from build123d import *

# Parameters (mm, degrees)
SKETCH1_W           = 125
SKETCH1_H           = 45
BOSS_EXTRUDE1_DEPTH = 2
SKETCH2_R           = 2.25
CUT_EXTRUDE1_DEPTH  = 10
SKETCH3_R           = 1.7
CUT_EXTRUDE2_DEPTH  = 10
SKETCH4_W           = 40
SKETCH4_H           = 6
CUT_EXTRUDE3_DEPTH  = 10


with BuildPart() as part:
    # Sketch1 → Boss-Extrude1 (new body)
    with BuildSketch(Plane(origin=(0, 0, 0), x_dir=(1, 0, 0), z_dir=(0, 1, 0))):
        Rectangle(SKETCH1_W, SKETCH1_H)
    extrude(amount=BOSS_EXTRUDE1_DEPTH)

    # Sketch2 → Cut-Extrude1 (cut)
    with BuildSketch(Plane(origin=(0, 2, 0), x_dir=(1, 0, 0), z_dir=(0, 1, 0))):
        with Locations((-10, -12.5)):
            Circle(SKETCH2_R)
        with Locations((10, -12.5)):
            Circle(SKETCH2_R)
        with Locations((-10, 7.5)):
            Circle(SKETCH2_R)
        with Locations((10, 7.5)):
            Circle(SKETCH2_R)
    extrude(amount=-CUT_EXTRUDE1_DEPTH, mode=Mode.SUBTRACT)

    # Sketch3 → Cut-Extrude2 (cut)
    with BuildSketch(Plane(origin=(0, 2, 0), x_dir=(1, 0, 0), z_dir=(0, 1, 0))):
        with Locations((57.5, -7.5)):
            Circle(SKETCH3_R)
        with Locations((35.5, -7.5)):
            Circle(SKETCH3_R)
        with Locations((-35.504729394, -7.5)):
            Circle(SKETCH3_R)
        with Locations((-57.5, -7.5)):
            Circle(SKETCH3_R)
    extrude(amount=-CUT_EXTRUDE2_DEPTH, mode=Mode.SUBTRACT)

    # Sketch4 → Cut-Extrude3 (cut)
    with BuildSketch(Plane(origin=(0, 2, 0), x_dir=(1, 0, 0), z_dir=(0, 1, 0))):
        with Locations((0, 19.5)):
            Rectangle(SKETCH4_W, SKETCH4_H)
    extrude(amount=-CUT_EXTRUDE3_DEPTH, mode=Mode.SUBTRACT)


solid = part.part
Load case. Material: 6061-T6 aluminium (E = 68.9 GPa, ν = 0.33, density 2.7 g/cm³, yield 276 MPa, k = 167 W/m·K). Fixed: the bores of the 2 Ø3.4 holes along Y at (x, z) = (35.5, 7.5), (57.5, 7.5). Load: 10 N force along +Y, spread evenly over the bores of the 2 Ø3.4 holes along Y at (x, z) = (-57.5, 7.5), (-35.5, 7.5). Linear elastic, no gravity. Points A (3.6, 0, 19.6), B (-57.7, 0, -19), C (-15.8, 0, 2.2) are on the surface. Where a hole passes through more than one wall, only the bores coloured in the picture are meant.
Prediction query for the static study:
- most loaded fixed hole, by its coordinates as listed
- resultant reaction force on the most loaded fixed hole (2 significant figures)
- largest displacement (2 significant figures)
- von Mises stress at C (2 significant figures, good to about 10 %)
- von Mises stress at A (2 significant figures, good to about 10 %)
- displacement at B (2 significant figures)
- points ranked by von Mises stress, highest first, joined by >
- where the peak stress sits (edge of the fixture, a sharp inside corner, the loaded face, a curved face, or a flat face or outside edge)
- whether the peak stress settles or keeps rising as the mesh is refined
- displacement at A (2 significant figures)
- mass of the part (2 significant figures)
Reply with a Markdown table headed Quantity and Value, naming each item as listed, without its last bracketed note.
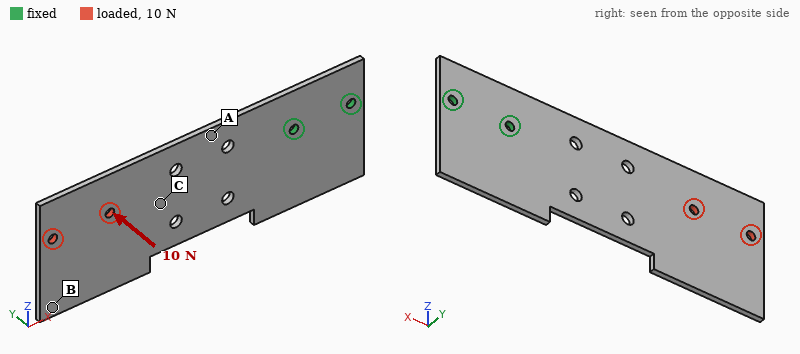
| Quantity | Value |
|---|---|
| most loaded fixed hole, by its coordinates as listed | (35.5, 7.5) |
| resultant reaction force on the most loaded fixed hole | 26 N |
| largest displacement | 1.4 mm |
| von Mises stress at C | 12 MPa |
| von Mises stress at A | 20 MPa |
| displacement at B | 1.3 mm |
| points ranked by von Mises stress, highest first, joined by > | A > C > B |
| where the peak stress sits | edge of the fixture |
| whether the peak stress settles or keeps rising as the mesh is refined | keeps rising |
| displacement at A | 0.21 mm |
| mass of the part | 29 g |
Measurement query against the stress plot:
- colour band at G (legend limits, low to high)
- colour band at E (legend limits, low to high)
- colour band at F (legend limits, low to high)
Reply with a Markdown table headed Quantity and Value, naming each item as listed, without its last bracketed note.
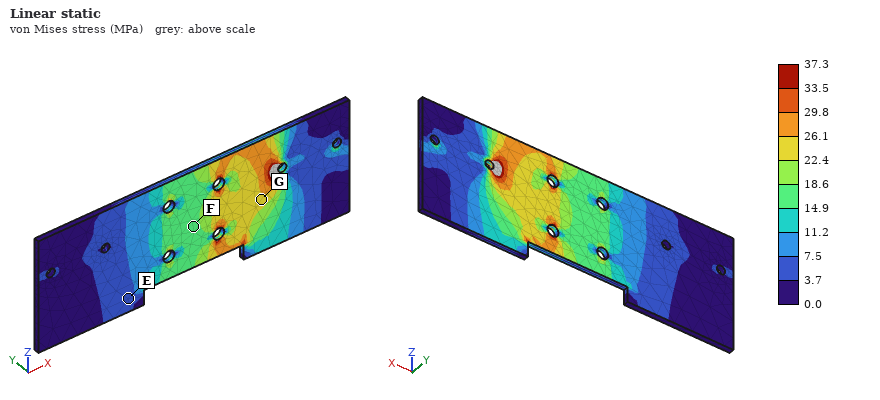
| Quantity | Value |
|---|---|
| colour band at G | 22.4 to 26.1 MPa |
| colour band at E | 3.7 to 7.5 MPa |
| colour band at F | 14.9 to 18.6 MPa |
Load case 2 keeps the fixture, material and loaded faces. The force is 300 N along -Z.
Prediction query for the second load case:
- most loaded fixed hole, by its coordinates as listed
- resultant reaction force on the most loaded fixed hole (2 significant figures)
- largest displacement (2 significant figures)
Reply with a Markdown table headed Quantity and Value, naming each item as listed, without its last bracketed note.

| Quantity | Value |
|---|---|
| most loaded fixed hole, by its coordinates as listed | (35.5, 7.5) |
| resultant reaction force on the most loaded fixed hole | 1.3 kN |
| largest displacement | 0.23 mm |
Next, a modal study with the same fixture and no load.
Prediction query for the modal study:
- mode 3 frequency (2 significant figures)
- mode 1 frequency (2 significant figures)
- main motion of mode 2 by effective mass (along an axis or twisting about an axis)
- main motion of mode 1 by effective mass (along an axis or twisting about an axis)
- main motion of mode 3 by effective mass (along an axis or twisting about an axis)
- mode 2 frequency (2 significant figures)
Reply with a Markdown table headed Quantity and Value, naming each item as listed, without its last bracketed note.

| Quantity | Value |
|---|---|
| mode 3 frequency | 1000 Hz |
| mode 1 frequency | 160 Hz |
| main motion of mode 2 by effective mass | twisting about X |
| main motion of mode 1 by effective mass | along Y |
| main motion of mode 3 by effective mass | along Y |
| mode 2 frequency | 660 Hz |
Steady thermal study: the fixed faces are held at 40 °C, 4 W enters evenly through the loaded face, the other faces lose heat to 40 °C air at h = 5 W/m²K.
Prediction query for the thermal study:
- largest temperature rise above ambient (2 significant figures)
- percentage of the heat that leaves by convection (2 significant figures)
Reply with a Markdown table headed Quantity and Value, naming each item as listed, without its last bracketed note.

| Quantity | Value |
|---|---|
| largest temperature rise above ambient | 26 K |
| percentage of the heat that leaves by convection | 16 % |
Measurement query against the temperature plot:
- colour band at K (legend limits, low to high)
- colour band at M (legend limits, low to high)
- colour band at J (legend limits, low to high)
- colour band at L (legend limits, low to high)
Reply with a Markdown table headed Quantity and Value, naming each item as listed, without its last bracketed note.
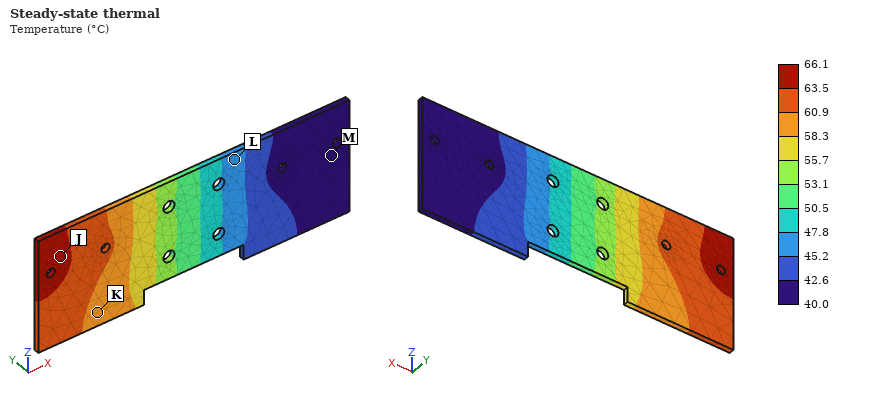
| Quantity | Value |
|---|---|
| colour band at K | 58.3 to 60.9 °C |
| colour band at M | 40.0 to 42.6 °C |
| colour band at J | 63.5 to 66.1 °C |
| colour band at L | 45.2 to 47.8 °C |
